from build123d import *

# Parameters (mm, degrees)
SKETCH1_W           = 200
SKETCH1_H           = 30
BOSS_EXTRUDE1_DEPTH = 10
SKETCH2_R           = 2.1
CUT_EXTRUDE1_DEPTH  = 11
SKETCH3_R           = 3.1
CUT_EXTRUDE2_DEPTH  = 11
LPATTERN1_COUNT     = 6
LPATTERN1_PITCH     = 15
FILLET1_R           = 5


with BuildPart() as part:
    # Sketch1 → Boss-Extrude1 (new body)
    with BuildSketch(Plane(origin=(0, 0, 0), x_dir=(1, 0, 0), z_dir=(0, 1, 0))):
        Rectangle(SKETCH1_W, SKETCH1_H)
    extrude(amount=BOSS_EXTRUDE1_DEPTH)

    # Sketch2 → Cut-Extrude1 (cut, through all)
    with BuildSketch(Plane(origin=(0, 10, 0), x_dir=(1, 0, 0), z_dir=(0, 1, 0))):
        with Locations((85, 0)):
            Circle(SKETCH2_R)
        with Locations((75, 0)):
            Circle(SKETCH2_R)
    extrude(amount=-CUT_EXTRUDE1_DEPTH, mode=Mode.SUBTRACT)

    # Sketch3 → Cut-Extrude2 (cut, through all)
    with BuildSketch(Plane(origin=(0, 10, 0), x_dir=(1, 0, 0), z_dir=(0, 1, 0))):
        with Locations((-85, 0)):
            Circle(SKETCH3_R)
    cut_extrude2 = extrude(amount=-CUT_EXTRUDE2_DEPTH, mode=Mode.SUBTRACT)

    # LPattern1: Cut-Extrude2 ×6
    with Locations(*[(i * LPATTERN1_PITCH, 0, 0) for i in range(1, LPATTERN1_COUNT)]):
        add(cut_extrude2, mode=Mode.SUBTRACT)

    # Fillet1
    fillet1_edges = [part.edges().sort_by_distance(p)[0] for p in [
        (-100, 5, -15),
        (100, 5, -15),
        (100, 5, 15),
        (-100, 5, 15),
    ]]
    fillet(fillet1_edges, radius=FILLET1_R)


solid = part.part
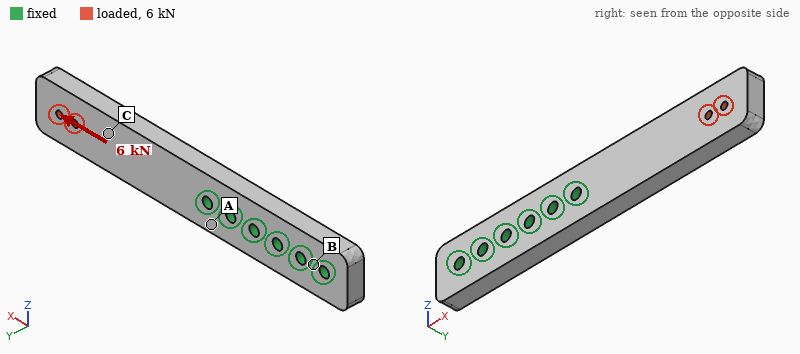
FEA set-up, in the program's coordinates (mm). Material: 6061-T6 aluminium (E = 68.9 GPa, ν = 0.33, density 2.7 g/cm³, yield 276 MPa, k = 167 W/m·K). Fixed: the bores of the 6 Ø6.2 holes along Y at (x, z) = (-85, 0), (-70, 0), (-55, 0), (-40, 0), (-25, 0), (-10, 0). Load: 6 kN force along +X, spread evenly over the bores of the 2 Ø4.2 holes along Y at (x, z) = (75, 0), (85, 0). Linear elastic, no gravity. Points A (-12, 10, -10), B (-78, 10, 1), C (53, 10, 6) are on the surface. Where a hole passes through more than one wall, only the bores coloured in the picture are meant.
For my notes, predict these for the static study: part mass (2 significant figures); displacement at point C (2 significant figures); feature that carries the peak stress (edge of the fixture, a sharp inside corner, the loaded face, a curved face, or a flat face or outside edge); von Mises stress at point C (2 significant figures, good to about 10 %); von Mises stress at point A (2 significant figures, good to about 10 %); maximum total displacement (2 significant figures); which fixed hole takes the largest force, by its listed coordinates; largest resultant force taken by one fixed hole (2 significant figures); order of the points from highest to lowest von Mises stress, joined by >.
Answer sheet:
160 g
20 µm
the loaded face
21 MPa
11 MPa
30 µm
(-10, 0)
4.5 kN
C > A > B
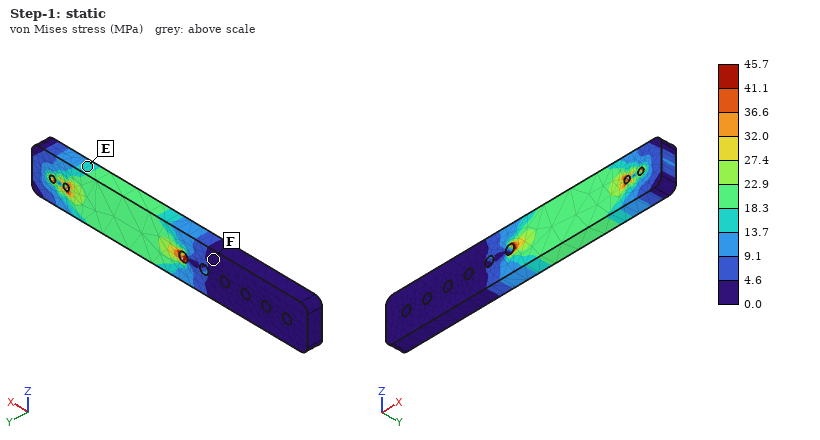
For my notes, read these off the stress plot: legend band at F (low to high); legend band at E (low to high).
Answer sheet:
0.0 to 4.6 MPa
13.7 to 18.3 MPa
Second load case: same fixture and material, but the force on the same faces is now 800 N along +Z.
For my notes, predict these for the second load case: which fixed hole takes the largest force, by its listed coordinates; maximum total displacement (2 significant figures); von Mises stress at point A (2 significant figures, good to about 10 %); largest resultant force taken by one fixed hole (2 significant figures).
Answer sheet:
(-10, 0)
0.24 mm
28 MPa
3.0 kN
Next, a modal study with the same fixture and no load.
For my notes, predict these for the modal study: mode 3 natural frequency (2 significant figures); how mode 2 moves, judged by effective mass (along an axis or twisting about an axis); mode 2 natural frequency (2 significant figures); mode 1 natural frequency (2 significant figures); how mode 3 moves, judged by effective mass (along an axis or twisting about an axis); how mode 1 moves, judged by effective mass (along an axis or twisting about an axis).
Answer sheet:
4000 Hz
along Z
1600 Hz
680 Hz
twisting about X
along Y
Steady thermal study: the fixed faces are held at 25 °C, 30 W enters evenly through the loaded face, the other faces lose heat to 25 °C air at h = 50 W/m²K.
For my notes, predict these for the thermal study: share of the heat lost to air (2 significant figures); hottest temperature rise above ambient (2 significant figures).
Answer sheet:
35 %
42 K
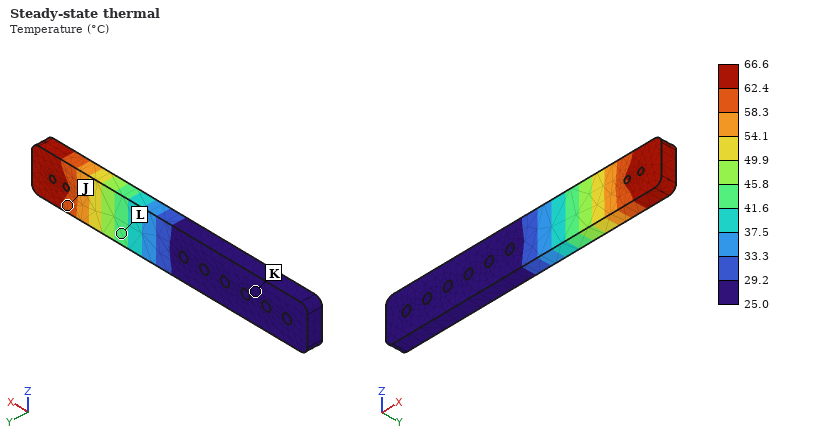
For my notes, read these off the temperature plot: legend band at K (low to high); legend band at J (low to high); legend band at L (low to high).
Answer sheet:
25.0 to 29.2 °C
58.3 to 62.4 °C
41.6 to 45.8 °C
